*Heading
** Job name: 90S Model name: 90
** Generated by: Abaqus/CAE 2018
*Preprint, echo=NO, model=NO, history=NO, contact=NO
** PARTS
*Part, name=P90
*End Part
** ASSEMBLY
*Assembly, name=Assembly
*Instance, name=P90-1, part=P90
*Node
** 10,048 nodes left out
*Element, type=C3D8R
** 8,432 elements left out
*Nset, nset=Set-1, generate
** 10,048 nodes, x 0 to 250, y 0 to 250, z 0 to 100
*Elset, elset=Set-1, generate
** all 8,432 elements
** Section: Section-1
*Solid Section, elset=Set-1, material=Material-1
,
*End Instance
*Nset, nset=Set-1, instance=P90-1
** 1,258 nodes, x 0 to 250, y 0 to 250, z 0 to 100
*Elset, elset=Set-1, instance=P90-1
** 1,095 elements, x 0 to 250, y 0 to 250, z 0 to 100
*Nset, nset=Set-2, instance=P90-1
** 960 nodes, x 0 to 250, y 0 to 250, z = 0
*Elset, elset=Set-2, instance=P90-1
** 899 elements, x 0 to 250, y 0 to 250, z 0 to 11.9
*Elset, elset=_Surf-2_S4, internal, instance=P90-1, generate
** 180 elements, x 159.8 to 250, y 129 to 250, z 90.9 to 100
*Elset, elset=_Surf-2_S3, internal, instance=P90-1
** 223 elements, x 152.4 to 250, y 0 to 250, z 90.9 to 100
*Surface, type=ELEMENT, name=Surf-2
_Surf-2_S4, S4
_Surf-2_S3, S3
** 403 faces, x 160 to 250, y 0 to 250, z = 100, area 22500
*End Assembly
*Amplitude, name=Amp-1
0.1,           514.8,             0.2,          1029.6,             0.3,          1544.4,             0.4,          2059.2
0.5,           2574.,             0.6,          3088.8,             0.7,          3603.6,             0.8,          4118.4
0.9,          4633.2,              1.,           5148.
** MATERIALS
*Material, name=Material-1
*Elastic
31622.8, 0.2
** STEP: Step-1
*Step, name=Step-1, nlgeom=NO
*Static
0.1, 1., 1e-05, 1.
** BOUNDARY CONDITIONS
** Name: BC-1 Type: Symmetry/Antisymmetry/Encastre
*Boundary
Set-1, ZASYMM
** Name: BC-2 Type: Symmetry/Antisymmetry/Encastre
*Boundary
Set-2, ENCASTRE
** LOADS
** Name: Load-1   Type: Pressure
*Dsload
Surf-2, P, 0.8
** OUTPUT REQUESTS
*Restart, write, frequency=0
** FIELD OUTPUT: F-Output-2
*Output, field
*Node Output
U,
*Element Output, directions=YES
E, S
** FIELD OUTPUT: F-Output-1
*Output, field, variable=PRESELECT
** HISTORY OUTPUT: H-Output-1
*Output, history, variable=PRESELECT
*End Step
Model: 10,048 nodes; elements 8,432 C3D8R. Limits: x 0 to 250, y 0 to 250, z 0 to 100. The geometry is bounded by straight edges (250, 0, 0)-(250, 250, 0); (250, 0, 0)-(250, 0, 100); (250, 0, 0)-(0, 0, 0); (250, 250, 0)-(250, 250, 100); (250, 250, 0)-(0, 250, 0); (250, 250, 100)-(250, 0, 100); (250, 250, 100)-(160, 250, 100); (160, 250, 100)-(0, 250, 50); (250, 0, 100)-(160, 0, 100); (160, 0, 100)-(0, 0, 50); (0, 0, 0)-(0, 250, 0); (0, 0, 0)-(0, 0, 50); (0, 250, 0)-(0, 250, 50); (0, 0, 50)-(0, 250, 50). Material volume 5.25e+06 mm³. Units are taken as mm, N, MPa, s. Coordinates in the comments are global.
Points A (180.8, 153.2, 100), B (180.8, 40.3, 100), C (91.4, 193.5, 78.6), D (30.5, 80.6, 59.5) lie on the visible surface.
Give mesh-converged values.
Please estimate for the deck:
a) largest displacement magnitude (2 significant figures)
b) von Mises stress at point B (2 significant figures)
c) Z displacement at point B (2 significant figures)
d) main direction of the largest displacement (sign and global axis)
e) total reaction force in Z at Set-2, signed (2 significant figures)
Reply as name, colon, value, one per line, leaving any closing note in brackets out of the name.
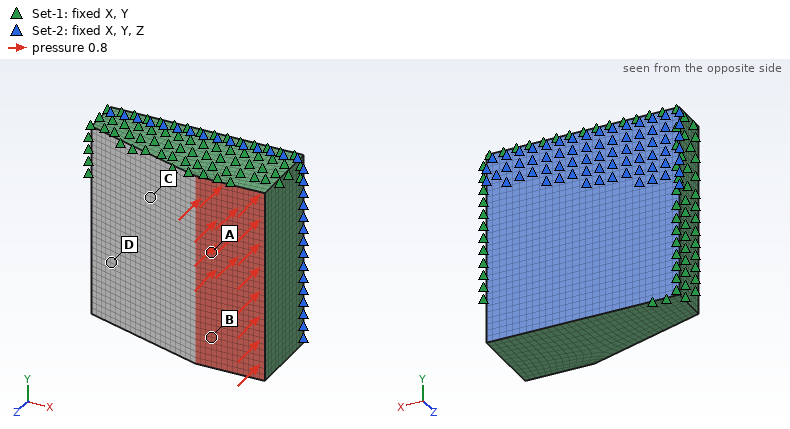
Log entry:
largest displacement magnitude: 0.0023 mm
von Mises stress at point B: 0.48 MPa
Z displacement at point B: -0.0018 mm
main direction of the largest displacement: -Z
total reaction force in Z at Set-2, signed: 18000 N
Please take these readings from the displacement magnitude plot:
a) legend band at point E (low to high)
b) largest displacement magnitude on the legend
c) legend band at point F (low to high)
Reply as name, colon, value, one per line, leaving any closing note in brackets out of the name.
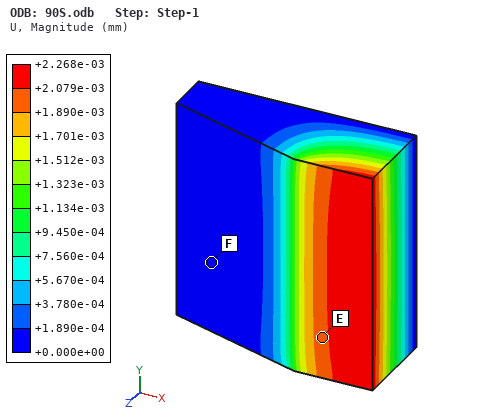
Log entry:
legend band at point E: +1.890e-03 to +2.079e-03 mm
largest displacement magnitude on the legend: +2.268e-03 mm
legend band at point F: +0.000e+00 to +1.890e-04 mm
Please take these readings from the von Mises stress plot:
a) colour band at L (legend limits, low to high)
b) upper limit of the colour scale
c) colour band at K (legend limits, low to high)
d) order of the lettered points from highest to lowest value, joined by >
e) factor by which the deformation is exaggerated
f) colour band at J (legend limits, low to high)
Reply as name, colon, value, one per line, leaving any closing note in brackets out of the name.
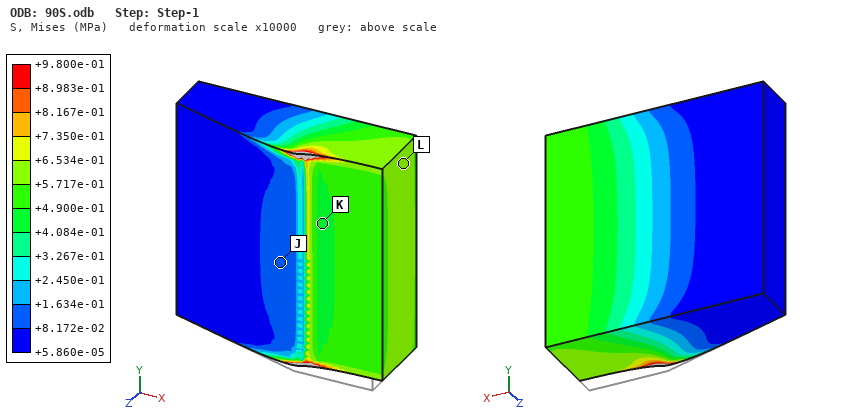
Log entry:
colour band at L: +5.717e-01 to +6.534e-01 MPa
upper limit of the colour scale: +9.800e-01 MPa
colour band at K: +4.084e-01 to +4.900e-01 MPa
order of the lettered points from highest to lowest value, joined by >: L > K > J
factor by which the deformation is exaggerated: 10000
colour band at J: +8.172e-02 to +1.634e-01 MPa
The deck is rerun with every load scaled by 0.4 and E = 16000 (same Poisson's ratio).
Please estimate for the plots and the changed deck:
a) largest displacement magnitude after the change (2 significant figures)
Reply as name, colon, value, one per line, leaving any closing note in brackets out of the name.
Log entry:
largest displacement magnitude after the change: 0.0018 mm
